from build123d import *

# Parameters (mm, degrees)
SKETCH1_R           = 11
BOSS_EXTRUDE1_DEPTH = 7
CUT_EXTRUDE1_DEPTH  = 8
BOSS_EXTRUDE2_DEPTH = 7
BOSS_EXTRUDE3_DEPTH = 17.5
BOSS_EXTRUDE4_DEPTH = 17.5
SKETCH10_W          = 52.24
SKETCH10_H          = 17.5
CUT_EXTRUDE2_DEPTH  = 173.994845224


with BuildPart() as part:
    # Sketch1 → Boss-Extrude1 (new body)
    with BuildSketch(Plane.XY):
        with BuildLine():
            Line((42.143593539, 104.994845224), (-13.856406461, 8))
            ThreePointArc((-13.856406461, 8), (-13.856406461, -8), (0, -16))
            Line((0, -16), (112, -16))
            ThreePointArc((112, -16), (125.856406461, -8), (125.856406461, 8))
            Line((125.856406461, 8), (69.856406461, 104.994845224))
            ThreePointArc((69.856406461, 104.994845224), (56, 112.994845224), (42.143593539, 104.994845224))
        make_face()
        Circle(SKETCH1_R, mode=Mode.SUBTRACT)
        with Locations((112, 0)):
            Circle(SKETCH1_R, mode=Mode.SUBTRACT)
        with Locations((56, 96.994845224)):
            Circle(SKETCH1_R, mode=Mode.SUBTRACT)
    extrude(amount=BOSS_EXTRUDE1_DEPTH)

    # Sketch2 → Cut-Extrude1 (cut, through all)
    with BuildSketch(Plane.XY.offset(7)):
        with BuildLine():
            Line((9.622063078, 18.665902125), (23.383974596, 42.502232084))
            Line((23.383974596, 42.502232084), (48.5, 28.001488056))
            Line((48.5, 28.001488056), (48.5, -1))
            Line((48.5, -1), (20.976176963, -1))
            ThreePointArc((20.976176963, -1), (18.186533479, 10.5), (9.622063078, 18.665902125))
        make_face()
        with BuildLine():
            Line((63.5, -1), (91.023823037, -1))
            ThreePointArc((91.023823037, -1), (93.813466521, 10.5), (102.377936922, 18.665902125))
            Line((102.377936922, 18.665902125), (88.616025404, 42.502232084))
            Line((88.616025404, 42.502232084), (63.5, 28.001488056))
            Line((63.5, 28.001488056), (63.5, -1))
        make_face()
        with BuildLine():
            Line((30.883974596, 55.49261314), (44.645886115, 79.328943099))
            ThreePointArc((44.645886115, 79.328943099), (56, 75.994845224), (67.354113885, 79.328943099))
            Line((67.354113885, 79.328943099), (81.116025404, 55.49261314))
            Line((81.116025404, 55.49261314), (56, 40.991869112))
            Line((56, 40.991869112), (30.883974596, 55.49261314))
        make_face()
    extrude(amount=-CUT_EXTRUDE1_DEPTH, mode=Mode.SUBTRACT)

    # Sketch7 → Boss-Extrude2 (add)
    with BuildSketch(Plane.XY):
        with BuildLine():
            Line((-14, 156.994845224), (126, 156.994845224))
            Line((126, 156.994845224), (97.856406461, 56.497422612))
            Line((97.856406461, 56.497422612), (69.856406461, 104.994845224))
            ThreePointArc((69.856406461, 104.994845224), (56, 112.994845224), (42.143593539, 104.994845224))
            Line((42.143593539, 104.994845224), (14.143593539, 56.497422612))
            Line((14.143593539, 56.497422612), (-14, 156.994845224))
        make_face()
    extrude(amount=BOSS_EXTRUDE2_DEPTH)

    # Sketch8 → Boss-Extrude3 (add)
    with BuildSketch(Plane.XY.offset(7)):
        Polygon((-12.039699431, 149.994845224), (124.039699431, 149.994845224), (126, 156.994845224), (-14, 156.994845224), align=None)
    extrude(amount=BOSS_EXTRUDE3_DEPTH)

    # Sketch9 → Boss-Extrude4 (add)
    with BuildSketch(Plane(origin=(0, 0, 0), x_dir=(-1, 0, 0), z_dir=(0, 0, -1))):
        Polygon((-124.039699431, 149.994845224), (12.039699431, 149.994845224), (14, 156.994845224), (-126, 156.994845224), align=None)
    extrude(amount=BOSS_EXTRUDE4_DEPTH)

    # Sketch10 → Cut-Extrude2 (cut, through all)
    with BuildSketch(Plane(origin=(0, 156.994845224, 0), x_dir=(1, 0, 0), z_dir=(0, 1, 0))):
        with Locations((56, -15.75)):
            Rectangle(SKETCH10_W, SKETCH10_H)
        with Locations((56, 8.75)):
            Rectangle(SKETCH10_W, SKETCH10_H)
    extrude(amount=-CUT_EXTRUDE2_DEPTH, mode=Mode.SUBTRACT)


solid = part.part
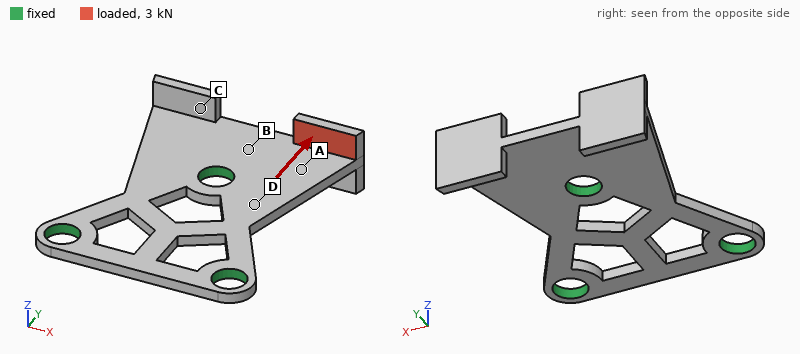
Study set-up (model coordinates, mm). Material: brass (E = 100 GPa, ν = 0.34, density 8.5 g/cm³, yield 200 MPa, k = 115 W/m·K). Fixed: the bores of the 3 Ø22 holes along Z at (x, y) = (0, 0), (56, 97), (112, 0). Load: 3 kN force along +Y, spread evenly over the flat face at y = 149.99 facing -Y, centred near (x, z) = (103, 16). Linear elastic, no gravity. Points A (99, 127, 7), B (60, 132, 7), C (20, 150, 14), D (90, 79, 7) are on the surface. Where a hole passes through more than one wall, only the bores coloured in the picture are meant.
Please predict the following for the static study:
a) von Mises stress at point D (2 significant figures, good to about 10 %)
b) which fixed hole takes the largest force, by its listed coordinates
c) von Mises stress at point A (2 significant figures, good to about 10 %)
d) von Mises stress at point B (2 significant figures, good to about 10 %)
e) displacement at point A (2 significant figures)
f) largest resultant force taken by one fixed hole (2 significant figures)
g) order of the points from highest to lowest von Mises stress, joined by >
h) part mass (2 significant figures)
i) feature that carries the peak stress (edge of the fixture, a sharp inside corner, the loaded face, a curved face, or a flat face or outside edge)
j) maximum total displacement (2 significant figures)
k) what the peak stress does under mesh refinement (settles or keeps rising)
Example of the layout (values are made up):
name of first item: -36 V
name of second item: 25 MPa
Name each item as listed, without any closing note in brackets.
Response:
von Mises stress at point D: 16 MPa
which fixed hole takes the largest force, by its listed coordinates: (56, 97)
von Mises stress at point A: 69 MPa
von Mises stress at point B: 42 MPa
displacement at point A: 0.075 mm
largest resultant force taken by one fixed hole: 2.5 kN
order of the points from highest to lowest von Mises stress, joined by >: A > B > D > C
part mass: 1.1 kg
feature that carries the peak stress: a sharp inside corner
maximum total displacement: 0.45 mm
what the peak stress does under mesh refinement: keeps rising
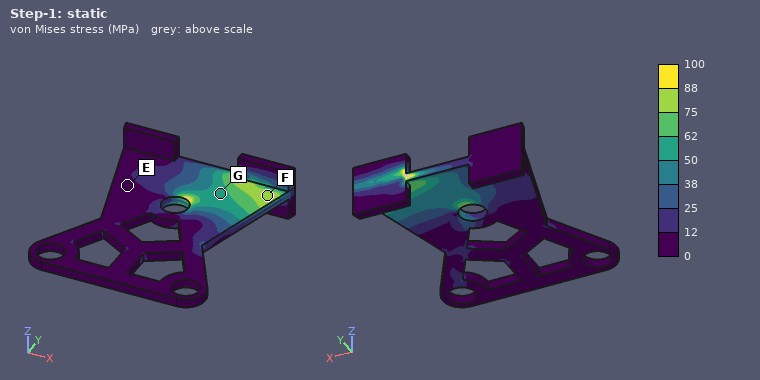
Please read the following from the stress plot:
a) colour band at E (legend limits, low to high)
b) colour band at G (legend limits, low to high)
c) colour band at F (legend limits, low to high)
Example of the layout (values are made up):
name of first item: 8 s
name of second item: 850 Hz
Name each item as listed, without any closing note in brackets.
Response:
colour band at E: 0 to 12 MPa
colour band at G: 50 to 62 MPa
colour band at F: 75 to 88 MPa
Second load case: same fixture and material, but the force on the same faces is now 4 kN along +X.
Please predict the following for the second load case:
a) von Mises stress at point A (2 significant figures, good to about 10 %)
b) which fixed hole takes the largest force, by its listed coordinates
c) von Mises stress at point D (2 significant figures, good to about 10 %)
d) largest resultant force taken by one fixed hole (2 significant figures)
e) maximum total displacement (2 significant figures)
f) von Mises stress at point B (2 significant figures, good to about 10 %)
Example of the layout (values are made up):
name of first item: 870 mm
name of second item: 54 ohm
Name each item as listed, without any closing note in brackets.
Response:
von Mises stress at point A: 73 MPa
which fixed hole takes the largest force, by its listed coordinates: (56, 97)
von Mises stress at point D: 32 MPa
largest resultant force taken by one fixed hole: 4.4 kN
maximum total displacement: 0.65 mm
von Mises stress at point B: 66 MPa
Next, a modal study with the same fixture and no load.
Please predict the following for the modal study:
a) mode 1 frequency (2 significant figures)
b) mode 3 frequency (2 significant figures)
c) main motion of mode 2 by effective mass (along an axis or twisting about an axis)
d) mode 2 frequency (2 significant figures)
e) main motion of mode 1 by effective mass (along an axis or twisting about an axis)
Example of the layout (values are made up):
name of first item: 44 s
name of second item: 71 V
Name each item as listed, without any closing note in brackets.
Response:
mode 1 frequency: 580 Hz
mode 3 frequency: 1500 Hz
main motion of mode 2 by effective mass: along Z
mode 2 frequency: 610 Hz
main motion of mode 1 by effective mass: twisting about Y
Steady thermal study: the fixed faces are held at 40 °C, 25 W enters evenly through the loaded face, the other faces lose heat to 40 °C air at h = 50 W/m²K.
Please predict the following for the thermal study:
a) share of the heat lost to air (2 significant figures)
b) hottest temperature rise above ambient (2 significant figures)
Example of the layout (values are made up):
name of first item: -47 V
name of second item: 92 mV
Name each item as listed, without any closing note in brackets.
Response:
share of the heat lost to air: 43 %
hottest temperature rise above ambient: 31 K
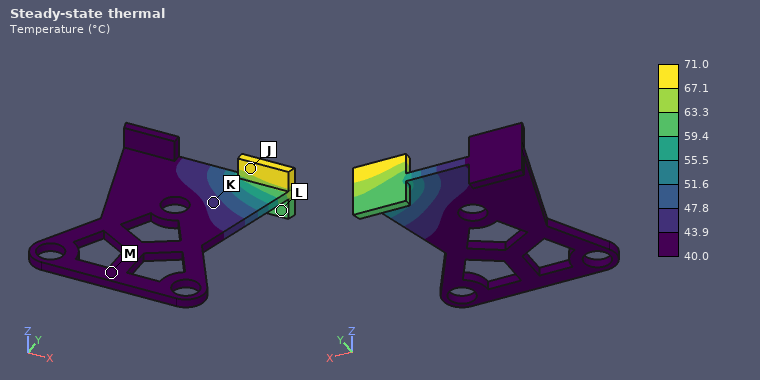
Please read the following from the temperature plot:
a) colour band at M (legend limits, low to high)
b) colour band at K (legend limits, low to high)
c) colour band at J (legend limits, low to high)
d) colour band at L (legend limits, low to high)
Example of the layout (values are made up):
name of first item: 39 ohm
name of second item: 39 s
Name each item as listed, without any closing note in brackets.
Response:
colour band at M: 40.0 to 43.9 °C
colour band at K: 43.9 to 47.8 °C
colour band at J: 67.1 to 71.0 °C
colour band at L: 59.4 to 63.3 °C
